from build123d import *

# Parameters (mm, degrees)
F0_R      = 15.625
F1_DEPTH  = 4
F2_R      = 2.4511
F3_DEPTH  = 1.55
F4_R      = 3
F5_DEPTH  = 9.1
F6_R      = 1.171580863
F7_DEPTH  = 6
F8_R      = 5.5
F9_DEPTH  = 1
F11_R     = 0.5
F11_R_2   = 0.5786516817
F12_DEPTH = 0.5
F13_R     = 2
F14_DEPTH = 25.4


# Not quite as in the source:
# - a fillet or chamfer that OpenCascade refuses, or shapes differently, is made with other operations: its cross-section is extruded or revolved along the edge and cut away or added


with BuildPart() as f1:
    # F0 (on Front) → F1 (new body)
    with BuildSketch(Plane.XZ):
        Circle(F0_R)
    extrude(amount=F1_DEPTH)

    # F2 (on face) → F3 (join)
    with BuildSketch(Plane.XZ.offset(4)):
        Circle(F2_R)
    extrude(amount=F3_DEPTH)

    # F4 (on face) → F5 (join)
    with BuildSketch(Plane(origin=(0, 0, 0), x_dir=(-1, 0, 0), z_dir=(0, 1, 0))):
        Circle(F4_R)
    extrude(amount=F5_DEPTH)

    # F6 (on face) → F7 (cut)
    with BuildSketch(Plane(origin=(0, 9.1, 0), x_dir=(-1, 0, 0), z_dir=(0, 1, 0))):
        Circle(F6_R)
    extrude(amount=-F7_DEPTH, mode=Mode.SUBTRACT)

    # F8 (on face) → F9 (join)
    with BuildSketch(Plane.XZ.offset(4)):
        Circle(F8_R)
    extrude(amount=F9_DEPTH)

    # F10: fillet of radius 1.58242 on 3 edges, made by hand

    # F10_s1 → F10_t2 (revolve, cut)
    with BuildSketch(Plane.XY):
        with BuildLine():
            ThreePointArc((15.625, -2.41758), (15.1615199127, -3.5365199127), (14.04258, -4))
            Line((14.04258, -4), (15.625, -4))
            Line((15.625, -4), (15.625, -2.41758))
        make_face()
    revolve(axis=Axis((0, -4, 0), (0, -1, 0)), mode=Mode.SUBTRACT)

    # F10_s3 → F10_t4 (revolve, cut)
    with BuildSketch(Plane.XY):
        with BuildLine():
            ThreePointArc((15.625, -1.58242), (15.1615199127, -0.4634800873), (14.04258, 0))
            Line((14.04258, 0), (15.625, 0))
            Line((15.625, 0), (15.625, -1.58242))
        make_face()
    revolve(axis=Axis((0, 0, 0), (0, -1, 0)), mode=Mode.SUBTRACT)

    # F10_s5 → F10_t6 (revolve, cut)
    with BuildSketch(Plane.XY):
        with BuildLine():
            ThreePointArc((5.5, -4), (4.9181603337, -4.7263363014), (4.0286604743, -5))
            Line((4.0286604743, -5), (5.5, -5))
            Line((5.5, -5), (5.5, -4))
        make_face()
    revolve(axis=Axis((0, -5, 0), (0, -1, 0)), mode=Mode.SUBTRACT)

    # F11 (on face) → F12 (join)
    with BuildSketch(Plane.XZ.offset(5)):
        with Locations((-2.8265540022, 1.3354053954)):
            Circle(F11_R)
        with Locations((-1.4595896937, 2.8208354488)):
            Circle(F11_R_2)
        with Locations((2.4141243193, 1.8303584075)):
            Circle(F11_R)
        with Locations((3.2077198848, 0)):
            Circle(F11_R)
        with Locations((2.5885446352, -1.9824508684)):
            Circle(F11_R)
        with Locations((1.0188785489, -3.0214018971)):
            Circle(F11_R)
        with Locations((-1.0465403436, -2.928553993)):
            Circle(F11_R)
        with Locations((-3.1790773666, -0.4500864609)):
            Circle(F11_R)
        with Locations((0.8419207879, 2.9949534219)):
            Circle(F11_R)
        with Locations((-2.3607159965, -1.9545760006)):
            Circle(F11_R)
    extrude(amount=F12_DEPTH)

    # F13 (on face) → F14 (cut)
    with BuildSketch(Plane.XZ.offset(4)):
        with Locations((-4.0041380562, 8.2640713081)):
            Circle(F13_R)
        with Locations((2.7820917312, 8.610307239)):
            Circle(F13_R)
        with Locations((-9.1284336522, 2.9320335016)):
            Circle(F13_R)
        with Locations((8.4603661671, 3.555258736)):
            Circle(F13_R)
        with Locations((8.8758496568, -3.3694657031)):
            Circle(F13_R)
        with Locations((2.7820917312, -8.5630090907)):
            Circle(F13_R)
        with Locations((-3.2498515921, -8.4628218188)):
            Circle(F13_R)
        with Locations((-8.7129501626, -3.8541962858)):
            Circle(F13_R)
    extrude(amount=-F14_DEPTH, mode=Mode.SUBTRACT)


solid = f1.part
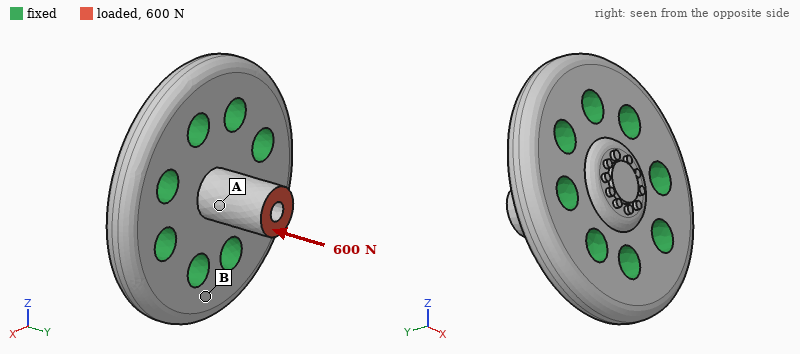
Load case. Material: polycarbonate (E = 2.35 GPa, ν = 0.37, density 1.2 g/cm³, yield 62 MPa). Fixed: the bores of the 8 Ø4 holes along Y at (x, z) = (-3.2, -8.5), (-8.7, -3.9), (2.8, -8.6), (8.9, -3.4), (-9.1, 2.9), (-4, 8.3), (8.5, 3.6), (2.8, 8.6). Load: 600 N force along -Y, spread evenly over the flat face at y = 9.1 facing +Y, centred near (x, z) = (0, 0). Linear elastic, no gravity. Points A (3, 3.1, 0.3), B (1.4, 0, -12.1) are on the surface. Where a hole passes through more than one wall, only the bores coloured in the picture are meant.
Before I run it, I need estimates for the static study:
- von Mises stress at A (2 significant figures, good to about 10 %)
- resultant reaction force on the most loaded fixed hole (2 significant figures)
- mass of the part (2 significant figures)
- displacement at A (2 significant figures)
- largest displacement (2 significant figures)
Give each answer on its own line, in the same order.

23 MPa
84 N
3.5 g
0.079 mm
0.14 mm
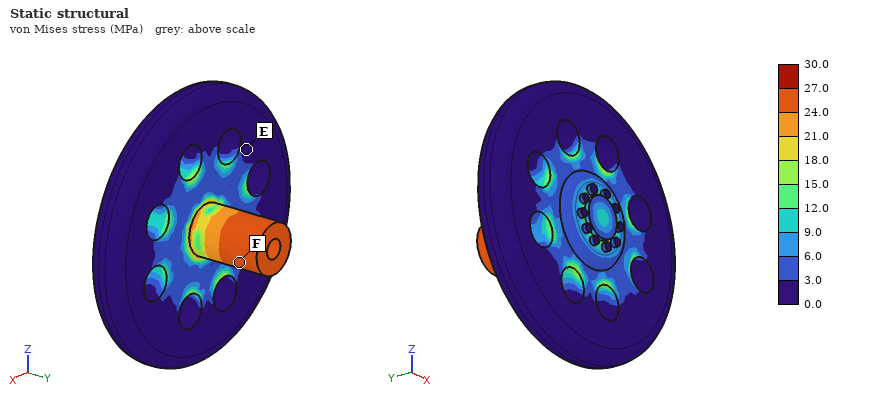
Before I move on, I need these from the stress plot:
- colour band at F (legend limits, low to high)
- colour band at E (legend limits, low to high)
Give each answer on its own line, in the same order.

24.0 to 27.0 MPa
0.0 to 3.0 MPa
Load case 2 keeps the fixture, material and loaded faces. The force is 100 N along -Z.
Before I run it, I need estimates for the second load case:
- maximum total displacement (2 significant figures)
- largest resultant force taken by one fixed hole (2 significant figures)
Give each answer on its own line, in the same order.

0.34 mm
50 N
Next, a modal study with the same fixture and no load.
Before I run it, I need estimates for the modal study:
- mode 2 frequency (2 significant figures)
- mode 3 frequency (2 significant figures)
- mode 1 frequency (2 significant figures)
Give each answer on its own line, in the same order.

9800 Hz
21 kHz
9700 Hz
